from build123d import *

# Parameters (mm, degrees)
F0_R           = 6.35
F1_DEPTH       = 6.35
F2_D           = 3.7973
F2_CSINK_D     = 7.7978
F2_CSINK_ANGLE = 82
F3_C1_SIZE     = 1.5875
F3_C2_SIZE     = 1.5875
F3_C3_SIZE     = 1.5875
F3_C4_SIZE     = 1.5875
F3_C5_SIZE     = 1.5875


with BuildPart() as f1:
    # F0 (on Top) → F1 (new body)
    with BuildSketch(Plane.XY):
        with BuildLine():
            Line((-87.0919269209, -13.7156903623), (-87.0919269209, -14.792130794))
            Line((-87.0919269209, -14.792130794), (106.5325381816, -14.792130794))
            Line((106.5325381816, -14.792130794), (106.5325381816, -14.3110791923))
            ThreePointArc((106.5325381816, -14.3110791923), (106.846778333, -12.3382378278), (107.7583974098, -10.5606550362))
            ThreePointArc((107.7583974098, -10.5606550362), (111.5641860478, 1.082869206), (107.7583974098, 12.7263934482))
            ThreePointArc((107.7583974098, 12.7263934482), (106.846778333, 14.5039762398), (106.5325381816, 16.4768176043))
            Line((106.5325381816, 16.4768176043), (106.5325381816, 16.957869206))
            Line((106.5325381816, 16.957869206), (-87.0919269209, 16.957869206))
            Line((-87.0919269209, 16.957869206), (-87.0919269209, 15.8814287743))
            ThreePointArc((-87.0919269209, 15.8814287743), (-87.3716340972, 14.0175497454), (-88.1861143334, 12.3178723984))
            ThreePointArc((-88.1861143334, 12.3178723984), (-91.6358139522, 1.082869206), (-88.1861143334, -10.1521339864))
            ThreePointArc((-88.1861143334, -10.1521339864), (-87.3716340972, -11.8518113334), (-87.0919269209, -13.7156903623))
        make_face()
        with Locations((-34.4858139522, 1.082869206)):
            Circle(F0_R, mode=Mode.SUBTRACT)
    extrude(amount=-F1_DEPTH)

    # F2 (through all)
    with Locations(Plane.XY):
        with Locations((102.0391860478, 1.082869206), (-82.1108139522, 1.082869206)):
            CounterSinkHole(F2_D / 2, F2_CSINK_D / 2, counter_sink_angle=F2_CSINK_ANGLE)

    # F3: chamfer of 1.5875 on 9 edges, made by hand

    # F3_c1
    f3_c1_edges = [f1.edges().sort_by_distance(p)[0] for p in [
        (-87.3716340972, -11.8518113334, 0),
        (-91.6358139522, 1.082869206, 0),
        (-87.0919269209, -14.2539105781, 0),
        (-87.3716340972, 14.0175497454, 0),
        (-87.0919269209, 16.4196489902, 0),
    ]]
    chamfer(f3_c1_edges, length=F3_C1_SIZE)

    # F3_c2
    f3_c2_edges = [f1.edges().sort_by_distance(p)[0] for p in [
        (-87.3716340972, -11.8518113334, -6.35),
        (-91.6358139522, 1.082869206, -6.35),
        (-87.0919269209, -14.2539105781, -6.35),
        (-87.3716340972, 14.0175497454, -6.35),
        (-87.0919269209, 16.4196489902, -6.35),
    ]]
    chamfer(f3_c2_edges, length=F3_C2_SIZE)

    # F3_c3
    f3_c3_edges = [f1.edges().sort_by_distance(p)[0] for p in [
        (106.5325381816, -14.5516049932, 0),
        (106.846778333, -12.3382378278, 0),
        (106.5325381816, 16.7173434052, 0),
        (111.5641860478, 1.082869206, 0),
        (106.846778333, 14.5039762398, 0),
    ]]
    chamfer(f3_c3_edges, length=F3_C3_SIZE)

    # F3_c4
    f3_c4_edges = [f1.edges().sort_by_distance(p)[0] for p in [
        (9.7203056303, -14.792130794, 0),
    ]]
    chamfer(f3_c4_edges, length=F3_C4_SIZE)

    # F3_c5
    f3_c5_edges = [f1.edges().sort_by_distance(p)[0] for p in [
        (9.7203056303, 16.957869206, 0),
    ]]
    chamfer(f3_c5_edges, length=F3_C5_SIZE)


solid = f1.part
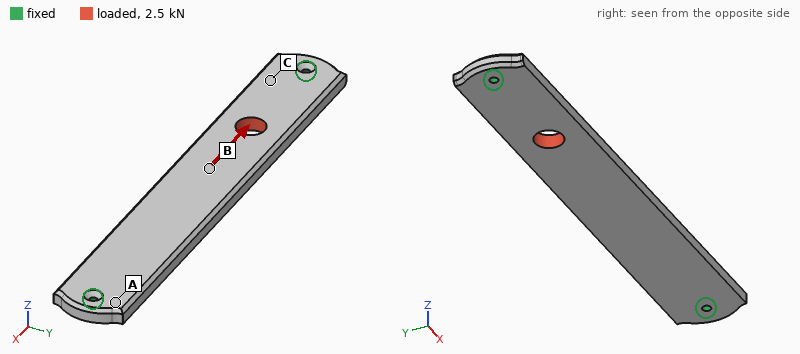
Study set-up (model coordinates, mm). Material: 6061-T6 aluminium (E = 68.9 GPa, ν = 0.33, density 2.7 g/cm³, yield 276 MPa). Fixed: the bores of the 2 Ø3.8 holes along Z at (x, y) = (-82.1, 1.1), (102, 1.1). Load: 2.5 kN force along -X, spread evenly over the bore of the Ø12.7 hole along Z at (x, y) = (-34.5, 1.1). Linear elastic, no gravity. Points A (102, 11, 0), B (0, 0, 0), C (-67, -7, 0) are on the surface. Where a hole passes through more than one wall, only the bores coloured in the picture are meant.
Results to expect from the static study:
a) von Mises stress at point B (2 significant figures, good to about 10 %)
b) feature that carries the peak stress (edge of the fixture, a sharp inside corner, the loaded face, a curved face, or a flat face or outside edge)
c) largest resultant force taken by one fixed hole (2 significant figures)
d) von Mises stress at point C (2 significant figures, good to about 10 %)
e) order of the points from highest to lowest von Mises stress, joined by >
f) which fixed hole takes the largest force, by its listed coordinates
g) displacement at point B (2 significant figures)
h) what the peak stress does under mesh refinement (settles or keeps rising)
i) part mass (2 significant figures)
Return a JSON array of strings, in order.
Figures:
["4.7 MPa", "edge of the fixture", "1.7 kN", "7.9 MPa", "C > B > A", "(-82.1, 1.1)", "9.4 µm", "keeps rising", "100 g"]
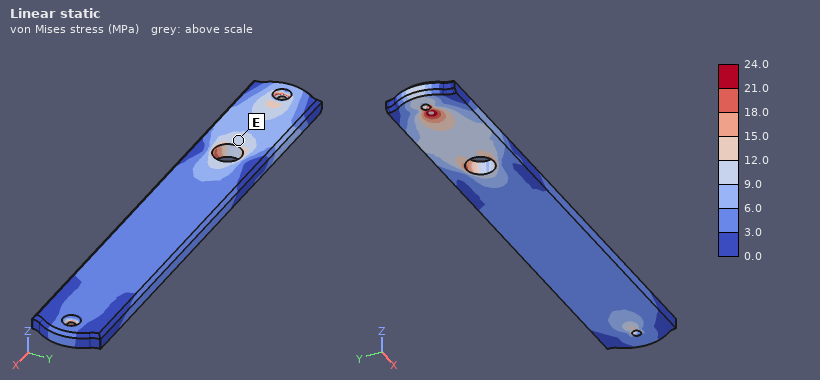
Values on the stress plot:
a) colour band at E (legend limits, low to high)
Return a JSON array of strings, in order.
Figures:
["9.0 to 12.0 MPa"]
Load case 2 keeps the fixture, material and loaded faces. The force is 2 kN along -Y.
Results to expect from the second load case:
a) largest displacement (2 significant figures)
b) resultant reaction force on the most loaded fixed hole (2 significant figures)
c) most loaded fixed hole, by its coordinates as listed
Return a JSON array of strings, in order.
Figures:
["0.14 mm", "1.5 kN", "(-82.1, 1.1)"]
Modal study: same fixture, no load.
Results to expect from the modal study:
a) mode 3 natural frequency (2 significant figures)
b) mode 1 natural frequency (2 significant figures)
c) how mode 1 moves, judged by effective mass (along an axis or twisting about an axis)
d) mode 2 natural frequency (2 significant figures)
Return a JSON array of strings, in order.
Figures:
["2300 Hz", "830 Hz", "along Z", "2300 Hz"]
